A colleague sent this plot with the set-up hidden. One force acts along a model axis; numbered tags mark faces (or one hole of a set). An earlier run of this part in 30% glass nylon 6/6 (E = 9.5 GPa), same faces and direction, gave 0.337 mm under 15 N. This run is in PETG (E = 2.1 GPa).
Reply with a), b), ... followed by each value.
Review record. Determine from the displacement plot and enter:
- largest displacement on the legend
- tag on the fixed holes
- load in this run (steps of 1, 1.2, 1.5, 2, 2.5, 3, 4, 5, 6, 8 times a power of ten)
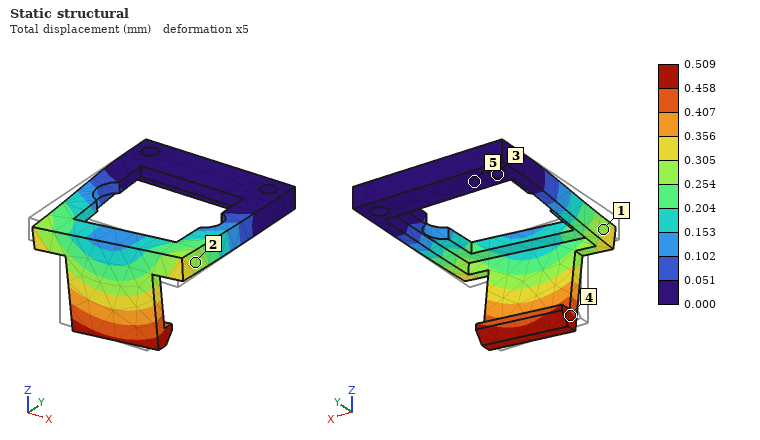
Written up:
a) 0.509 mm
b) 3
c) 5 N
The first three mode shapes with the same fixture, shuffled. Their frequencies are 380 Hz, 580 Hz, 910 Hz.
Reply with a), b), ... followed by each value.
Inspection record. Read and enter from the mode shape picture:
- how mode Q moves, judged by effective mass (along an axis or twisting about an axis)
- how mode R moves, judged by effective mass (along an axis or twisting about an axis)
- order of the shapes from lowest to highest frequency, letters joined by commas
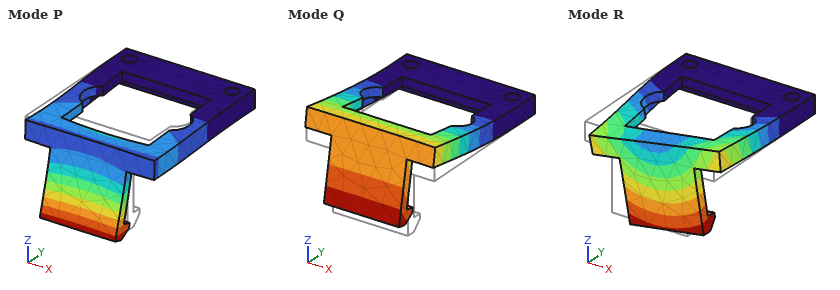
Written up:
a) along Z
b) along X
c) Q, R, P
